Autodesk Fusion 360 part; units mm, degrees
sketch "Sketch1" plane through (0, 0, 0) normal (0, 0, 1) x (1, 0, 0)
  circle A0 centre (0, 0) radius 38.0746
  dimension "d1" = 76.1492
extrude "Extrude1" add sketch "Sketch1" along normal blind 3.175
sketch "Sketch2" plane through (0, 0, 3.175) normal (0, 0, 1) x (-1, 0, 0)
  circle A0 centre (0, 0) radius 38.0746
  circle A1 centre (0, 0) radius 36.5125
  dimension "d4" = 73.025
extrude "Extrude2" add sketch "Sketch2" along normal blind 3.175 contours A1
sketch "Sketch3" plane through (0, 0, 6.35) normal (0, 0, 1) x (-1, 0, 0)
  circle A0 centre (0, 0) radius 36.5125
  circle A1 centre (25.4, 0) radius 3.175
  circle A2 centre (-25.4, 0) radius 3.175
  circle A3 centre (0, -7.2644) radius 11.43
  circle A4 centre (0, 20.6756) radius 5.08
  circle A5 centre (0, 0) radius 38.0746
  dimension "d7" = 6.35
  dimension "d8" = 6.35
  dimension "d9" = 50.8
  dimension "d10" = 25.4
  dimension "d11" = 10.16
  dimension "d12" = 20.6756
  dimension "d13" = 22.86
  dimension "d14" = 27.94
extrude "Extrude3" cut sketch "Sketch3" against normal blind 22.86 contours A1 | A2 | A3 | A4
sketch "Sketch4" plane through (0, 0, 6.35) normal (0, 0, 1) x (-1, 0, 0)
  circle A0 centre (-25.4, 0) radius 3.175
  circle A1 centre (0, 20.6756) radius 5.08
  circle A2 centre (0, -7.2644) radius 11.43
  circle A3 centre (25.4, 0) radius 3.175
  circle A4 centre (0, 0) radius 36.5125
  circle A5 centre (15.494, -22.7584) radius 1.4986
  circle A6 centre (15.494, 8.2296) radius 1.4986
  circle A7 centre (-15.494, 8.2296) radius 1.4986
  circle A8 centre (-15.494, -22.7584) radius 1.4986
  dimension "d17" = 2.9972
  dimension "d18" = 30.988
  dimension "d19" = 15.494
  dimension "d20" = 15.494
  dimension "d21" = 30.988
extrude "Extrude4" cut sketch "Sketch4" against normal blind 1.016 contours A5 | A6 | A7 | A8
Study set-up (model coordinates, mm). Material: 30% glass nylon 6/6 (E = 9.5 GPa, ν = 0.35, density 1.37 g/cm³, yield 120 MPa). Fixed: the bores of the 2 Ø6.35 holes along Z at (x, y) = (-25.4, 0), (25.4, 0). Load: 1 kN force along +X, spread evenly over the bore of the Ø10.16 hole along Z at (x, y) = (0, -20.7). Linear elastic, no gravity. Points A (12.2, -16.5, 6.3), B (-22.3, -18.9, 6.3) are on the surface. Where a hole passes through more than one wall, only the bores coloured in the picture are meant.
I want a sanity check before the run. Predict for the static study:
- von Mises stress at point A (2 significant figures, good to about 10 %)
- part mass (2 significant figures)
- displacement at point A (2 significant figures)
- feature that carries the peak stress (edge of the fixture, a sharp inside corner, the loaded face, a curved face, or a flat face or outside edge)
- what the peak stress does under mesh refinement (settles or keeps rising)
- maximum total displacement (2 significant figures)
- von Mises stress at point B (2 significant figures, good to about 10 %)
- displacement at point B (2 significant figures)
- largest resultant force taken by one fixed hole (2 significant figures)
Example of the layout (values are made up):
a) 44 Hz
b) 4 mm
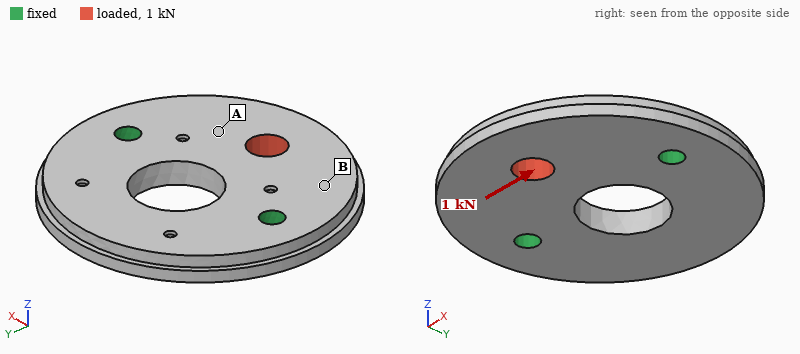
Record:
a) 5.0 MPa
b) 33 g
c) 17 µm
d) edge of the fixture
e) keeps rising
f) 29 µm
g) 2.3 MPa
h) 17 µm
i) 610 N
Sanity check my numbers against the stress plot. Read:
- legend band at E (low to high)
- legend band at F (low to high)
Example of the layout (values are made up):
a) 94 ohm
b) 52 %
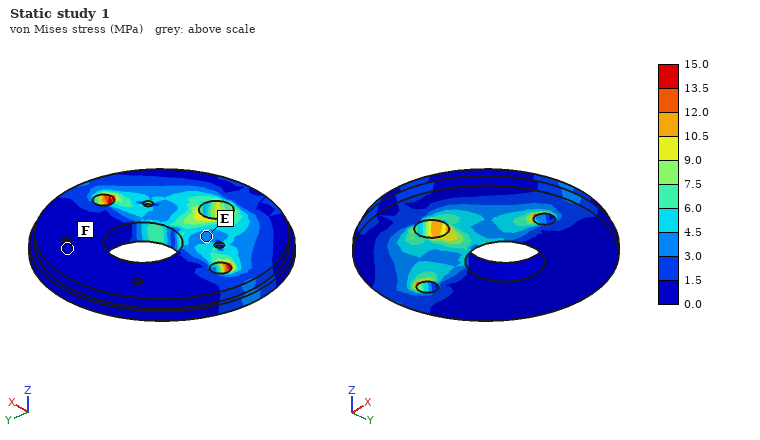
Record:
a) 3.0 to 4.5 MPa
b) 0.0 to 1.5 MPa
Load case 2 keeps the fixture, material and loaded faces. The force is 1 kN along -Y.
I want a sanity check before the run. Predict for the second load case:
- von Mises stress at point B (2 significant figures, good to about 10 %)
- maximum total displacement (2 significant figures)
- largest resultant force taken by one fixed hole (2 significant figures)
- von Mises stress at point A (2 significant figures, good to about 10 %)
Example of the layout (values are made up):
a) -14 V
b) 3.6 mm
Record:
a) 2.3 MPa
b) 22 µm
c) 550 N
d) 4.1 MPa
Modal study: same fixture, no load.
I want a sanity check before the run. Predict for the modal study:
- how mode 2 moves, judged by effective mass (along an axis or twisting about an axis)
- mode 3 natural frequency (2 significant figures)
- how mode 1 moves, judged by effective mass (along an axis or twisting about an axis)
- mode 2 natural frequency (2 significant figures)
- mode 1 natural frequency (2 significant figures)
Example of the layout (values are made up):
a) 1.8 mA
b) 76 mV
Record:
a) along Z
b) 4700 Hz
c) twisting about X
d) 2200 Hz
e) 2000 Hz
